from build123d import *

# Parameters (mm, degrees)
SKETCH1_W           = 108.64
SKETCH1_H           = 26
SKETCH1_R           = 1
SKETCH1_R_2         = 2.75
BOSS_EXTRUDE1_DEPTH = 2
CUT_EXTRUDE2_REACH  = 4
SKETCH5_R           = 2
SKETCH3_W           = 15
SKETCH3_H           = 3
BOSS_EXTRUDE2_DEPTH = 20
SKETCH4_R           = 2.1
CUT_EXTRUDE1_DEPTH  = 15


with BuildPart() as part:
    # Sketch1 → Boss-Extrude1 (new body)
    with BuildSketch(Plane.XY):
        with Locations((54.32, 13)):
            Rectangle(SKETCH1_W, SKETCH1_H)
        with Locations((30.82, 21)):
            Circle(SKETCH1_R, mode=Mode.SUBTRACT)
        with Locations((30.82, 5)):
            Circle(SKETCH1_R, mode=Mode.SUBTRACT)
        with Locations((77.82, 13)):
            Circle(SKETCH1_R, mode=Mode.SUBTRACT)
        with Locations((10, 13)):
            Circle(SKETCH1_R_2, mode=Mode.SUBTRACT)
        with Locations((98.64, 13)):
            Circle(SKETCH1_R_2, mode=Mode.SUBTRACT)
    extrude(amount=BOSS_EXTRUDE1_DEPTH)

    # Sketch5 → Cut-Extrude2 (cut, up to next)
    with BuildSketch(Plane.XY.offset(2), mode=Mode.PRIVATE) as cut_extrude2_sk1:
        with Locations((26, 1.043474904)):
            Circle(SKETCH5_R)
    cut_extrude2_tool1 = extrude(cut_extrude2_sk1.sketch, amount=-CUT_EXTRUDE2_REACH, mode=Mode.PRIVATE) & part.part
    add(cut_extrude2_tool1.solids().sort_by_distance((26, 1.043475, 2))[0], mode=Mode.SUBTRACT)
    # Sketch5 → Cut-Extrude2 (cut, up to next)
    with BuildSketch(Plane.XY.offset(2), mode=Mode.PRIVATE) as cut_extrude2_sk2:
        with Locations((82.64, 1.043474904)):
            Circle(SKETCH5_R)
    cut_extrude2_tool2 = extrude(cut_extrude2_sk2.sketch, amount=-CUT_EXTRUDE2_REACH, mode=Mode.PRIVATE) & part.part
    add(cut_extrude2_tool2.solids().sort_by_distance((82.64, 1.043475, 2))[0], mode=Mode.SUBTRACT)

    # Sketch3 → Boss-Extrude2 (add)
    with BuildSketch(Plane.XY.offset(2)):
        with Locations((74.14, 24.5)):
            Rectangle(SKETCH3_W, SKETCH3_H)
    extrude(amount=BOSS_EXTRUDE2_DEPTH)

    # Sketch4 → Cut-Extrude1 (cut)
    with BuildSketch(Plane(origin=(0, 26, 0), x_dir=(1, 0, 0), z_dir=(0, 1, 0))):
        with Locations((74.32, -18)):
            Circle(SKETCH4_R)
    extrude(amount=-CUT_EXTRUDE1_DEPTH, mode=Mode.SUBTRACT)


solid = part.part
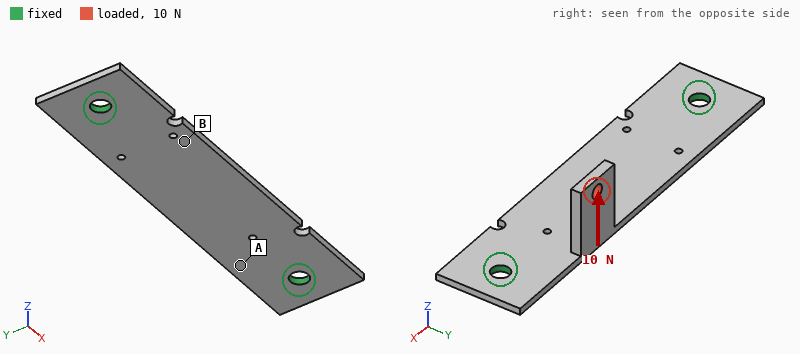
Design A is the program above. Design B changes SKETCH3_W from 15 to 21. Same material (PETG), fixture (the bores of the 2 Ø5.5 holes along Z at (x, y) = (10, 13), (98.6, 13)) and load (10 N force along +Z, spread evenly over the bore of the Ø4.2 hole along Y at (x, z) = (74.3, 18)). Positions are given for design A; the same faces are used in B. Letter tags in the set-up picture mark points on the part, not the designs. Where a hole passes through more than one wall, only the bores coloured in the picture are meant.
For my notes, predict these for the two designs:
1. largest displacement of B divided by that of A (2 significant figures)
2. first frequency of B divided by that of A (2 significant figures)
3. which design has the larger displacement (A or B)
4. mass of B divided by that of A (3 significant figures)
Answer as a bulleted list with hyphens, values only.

- 0.92
- 0.96
- A
- 1.06
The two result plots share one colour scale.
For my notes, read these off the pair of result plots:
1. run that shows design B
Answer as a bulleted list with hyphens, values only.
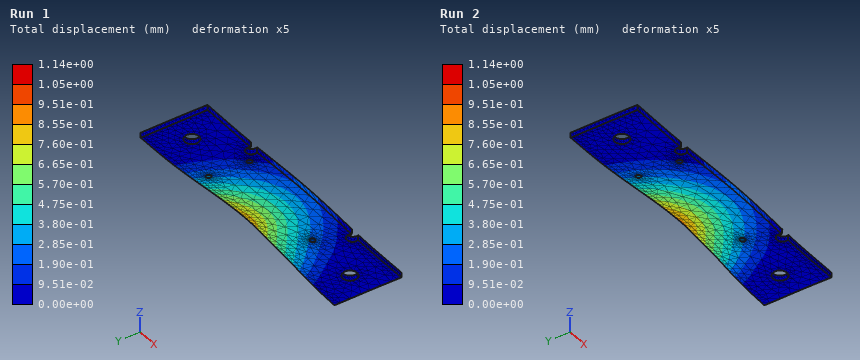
- Run 1
